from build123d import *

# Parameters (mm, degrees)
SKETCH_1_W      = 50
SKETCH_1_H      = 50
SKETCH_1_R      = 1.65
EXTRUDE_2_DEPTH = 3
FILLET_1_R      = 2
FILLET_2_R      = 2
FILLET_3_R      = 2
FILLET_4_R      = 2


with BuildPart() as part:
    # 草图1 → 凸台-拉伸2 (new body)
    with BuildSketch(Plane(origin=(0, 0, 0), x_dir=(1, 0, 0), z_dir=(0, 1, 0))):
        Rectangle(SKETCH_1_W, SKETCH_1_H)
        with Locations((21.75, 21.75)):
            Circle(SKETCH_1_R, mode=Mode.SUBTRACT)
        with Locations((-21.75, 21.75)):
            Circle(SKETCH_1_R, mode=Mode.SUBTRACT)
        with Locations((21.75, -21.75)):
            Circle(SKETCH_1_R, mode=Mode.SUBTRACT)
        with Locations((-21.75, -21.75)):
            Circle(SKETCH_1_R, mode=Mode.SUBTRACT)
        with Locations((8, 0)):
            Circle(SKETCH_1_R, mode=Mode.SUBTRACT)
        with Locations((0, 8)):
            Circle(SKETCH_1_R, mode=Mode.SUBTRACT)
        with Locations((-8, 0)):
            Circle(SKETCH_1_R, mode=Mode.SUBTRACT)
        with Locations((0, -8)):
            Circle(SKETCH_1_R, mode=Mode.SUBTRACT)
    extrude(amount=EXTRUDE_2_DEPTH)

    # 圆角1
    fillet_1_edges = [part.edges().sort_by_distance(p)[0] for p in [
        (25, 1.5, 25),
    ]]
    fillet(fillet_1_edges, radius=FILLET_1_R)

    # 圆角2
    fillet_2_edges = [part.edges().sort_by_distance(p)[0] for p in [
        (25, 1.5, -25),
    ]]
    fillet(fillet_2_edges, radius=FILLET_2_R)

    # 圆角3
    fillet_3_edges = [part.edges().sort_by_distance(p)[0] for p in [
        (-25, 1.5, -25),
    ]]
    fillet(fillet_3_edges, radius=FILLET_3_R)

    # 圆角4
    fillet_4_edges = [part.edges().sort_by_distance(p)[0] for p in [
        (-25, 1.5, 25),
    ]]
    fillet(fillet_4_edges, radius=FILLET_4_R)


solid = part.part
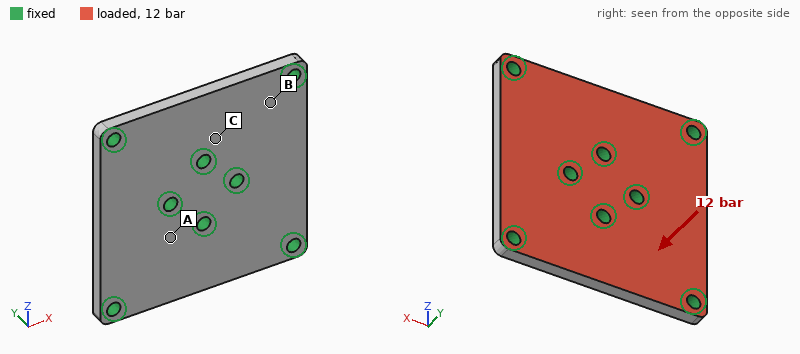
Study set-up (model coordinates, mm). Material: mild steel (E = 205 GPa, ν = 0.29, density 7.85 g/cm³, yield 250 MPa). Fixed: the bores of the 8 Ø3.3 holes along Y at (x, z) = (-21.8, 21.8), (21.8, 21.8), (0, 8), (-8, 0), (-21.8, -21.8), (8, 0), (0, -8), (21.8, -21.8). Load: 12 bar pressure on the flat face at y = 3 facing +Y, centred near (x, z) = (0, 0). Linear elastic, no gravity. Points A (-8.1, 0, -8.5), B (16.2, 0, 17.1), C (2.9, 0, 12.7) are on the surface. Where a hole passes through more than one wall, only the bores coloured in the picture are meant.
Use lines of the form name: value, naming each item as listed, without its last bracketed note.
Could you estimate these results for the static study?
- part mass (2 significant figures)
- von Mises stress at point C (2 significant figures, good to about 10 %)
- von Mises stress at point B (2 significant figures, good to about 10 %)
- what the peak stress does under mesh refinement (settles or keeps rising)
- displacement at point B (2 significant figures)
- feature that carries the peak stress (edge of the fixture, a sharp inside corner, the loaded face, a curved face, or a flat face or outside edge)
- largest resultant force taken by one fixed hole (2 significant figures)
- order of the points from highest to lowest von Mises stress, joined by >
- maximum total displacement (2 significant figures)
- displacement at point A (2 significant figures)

part mass: 57 g
von Mises stress at point C: 21 MPa
von Mises stress at point B: 31 MPa
what the peak stress does under mesh refinement: keeps rising
displacement at point B: 2.7 µm
feature that carries the peak stress: edge of the fixture
largest resultant force taken by one fixed hole: 400 N
order of the points from highest to lowest von Mises stress, joined by >: B > C > A
maximum total displacement: 10 µm
displacement at point A: 1.8 µm
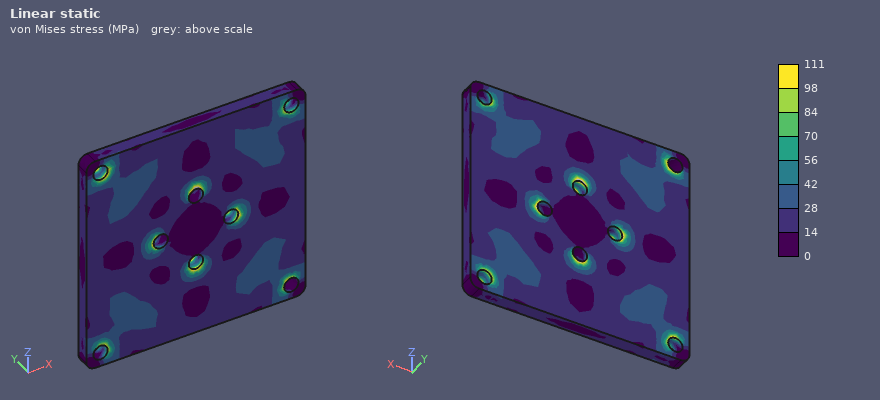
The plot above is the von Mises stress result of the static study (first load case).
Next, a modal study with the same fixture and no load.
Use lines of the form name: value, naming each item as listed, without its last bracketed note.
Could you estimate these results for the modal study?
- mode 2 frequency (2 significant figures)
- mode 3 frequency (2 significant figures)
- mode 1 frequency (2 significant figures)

mode 2 frequency: 14 kHz
mode 3 frequency: 14 kHz
mode 1 frequency: 13 kHz
